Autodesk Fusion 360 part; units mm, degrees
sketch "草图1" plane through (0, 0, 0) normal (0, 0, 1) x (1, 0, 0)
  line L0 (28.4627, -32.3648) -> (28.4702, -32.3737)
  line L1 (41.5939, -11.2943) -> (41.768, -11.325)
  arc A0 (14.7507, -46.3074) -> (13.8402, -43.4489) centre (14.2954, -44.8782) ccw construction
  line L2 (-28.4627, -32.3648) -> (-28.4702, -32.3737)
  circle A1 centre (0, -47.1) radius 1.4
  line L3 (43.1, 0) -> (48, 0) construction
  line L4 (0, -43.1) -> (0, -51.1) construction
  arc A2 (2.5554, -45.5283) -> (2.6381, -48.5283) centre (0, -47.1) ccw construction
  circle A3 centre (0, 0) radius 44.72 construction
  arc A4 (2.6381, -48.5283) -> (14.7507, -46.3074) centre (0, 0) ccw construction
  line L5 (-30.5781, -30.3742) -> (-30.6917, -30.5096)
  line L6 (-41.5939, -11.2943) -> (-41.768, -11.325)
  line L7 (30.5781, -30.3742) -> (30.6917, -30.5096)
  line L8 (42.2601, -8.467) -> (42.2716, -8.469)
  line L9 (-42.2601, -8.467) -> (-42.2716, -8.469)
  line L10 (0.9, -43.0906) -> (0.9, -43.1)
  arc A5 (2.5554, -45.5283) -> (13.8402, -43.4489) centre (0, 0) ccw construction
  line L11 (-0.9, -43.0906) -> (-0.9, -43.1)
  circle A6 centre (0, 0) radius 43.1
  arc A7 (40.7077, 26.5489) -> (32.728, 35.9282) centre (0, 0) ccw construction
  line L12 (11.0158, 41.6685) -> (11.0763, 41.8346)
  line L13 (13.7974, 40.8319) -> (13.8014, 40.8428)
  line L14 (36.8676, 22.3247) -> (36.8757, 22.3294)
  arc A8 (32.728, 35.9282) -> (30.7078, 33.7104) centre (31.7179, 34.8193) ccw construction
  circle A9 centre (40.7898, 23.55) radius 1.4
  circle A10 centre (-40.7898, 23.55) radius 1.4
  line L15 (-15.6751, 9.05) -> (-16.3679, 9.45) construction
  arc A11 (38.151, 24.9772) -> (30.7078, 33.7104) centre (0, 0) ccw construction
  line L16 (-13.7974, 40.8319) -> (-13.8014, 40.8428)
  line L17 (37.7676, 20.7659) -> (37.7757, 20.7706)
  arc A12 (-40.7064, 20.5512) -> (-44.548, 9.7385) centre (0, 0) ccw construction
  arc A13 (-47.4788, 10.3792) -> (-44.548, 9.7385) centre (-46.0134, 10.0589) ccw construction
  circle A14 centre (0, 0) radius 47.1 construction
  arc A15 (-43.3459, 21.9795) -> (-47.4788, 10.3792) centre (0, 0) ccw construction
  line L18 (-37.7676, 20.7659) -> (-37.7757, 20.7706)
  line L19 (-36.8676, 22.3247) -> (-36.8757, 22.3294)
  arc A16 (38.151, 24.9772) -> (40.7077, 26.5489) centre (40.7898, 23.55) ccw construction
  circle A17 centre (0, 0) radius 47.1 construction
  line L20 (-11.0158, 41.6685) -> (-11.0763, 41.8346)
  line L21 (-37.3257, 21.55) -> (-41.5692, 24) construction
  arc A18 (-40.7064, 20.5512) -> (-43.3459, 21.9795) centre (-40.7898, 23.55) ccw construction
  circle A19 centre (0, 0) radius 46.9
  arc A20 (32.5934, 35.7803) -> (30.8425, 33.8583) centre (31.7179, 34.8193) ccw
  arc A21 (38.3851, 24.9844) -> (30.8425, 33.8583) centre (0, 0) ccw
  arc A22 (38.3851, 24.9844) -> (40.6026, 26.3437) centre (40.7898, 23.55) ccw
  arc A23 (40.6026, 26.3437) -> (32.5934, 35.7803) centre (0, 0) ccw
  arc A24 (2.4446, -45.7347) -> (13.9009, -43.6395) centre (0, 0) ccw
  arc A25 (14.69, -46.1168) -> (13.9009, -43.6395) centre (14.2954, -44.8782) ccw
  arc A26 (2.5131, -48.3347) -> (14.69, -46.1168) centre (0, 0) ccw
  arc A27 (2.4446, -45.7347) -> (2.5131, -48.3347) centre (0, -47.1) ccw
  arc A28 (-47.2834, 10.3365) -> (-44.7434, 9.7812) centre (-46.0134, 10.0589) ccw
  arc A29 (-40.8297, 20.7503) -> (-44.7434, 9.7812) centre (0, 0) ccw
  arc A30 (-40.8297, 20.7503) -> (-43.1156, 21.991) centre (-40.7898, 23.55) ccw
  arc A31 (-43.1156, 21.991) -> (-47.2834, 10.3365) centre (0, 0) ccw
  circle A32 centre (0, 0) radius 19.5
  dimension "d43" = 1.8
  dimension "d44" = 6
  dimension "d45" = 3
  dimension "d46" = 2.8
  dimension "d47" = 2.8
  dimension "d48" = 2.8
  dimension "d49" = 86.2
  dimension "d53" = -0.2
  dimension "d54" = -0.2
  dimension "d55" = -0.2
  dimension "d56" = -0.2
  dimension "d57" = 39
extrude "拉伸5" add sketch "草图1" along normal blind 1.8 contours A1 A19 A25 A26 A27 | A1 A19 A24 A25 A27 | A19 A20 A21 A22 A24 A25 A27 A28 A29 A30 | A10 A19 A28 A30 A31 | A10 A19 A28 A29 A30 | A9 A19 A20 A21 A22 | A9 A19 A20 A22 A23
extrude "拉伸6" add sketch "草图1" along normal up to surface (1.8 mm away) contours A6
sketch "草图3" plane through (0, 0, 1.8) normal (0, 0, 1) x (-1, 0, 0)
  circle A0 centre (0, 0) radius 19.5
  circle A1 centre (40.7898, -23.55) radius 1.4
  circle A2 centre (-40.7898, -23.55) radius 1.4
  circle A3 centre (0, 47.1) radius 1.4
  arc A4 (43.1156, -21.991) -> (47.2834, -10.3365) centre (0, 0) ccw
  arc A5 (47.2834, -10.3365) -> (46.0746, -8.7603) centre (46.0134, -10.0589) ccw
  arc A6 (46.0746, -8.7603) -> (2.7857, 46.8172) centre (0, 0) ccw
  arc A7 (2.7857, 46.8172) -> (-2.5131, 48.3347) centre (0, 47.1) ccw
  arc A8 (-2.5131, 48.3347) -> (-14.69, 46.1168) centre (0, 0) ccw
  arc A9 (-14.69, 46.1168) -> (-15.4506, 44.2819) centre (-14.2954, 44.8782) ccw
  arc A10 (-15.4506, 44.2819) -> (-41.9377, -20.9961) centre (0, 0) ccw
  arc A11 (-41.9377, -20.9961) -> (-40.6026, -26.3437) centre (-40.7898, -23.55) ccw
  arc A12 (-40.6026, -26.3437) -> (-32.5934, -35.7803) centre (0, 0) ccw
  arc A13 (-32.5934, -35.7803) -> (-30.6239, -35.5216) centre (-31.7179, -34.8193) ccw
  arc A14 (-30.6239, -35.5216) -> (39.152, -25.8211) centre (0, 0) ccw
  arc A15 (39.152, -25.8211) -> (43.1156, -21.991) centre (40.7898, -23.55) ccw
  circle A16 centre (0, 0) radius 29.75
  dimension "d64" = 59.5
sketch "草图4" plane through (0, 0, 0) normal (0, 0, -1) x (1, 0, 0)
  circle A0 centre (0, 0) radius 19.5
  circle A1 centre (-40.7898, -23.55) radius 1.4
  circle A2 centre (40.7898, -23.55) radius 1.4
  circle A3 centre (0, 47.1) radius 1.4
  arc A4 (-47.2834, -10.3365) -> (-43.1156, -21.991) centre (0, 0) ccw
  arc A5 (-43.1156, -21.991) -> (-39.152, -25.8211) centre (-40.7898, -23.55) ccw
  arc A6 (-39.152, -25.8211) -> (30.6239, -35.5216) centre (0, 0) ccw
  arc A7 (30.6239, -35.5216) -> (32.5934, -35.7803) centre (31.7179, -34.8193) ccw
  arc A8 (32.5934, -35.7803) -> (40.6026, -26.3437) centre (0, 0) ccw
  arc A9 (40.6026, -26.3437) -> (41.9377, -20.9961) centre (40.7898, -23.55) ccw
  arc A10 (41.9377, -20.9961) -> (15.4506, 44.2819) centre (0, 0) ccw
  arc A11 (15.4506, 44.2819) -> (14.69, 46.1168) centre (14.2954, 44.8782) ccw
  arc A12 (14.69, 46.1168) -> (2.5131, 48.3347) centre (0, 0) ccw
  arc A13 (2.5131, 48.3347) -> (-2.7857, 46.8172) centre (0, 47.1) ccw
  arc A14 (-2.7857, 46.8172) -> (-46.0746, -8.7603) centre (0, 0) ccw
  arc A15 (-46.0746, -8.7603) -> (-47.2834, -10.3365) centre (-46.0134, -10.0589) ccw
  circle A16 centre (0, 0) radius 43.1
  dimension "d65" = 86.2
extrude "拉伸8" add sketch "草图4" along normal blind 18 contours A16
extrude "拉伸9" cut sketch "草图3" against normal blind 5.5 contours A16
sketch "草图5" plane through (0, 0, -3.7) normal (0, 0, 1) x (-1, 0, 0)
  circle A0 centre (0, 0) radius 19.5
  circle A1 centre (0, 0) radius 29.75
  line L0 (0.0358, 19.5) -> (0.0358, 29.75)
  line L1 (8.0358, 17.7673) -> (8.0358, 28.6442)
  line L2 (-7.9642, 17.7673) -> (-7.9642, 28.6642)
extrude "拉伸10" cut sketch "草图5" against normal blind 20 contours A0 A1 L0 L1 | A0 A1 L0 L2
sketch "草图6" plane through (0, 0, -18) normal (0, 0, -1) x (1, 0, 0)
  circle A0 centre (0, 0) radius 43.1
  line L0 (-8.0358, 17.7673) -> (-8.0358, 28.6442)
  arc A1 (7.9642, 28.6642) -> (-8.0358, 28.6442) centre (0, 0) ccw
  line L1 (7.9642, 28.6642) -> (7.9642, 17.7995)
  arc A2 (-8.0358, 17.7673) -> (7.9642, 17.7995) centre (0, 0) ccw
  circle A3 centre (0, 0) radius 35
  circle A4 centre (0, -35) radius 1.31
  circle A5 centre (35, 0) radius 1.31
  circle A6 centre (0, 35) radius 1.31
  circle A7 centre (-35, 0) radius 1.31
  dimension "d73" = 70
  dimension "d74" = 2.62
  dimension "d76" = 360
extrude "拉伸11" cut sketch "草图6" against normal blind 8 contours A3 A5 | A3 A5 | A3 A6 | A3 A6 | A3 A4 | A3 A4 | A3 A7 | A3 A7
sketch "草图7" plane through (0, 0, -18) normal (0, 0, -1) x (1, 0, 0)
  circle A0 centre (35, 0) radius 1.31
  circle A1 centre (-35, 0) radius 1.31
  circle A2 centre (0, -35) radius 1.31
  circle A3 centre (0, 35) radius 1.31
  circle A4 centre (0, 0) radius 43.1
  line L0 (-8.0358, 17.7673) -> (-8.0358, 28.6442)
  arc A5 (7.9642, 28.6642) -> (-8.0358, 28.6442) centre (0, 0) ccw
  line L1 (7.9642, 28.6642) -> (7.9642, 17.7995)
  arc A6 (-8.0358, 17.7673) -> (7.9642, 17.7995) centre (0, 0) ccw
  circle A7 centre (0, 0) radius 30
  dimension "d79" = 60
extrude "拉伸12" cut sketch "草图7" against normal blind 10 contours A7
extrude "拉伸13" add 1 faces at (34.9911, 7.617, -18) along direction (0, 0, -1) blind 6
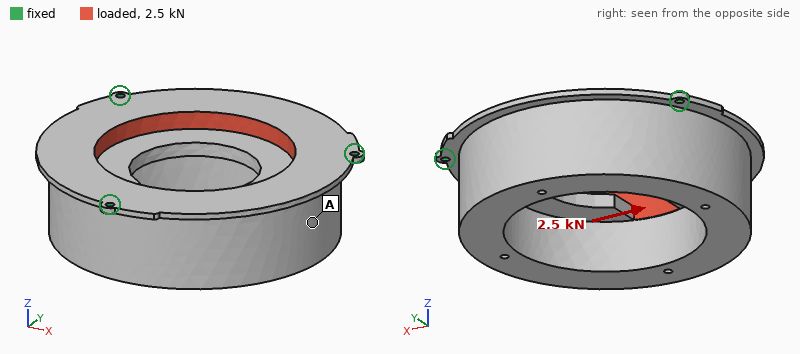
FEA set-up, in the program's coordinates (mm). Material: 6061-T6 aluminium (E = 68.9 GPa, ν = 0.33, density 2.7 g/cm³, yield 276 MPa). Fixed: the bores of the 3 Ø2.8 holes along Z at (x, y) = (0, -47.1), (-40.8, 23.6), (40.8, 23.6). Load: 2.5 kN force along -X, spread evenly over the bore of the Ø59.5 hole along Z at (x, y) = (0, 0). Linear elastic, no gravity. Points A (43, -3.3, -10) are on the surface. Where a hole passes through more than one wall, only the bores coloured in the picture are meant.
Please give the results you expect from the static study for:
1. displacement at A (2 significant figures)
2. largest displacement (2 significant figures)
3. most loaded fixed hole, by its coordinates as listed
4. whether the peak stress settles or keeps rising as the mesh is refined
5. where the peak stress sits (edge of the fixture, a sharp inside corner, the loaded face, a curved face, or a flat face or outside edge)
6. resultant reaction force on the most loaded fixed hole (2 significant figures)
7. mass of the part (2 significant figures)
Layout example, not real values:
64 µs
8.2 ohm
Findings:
8.8 µm
12 µm
(0, -47.1)
keeps rising
edge of the fixture
950 N
230 g
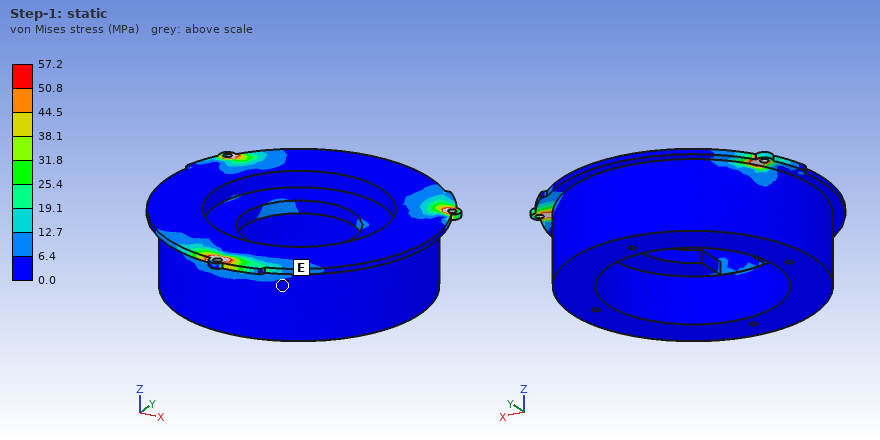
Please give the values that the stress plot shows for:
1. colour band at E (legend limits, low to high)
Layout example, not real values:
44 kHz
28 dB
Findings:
0.0 to 6.4 MPa
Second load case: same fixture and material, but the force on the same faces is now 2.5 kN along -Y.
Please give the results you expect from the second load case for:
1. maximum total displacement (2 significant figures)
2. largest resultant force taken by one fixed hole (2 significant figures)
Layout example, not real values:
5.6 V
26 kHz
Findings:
12 µm
870 N
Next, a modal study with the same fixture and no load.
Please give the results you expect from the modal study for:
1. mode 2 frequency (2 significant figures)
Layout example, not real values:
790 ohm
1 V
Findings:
3100 Hz
